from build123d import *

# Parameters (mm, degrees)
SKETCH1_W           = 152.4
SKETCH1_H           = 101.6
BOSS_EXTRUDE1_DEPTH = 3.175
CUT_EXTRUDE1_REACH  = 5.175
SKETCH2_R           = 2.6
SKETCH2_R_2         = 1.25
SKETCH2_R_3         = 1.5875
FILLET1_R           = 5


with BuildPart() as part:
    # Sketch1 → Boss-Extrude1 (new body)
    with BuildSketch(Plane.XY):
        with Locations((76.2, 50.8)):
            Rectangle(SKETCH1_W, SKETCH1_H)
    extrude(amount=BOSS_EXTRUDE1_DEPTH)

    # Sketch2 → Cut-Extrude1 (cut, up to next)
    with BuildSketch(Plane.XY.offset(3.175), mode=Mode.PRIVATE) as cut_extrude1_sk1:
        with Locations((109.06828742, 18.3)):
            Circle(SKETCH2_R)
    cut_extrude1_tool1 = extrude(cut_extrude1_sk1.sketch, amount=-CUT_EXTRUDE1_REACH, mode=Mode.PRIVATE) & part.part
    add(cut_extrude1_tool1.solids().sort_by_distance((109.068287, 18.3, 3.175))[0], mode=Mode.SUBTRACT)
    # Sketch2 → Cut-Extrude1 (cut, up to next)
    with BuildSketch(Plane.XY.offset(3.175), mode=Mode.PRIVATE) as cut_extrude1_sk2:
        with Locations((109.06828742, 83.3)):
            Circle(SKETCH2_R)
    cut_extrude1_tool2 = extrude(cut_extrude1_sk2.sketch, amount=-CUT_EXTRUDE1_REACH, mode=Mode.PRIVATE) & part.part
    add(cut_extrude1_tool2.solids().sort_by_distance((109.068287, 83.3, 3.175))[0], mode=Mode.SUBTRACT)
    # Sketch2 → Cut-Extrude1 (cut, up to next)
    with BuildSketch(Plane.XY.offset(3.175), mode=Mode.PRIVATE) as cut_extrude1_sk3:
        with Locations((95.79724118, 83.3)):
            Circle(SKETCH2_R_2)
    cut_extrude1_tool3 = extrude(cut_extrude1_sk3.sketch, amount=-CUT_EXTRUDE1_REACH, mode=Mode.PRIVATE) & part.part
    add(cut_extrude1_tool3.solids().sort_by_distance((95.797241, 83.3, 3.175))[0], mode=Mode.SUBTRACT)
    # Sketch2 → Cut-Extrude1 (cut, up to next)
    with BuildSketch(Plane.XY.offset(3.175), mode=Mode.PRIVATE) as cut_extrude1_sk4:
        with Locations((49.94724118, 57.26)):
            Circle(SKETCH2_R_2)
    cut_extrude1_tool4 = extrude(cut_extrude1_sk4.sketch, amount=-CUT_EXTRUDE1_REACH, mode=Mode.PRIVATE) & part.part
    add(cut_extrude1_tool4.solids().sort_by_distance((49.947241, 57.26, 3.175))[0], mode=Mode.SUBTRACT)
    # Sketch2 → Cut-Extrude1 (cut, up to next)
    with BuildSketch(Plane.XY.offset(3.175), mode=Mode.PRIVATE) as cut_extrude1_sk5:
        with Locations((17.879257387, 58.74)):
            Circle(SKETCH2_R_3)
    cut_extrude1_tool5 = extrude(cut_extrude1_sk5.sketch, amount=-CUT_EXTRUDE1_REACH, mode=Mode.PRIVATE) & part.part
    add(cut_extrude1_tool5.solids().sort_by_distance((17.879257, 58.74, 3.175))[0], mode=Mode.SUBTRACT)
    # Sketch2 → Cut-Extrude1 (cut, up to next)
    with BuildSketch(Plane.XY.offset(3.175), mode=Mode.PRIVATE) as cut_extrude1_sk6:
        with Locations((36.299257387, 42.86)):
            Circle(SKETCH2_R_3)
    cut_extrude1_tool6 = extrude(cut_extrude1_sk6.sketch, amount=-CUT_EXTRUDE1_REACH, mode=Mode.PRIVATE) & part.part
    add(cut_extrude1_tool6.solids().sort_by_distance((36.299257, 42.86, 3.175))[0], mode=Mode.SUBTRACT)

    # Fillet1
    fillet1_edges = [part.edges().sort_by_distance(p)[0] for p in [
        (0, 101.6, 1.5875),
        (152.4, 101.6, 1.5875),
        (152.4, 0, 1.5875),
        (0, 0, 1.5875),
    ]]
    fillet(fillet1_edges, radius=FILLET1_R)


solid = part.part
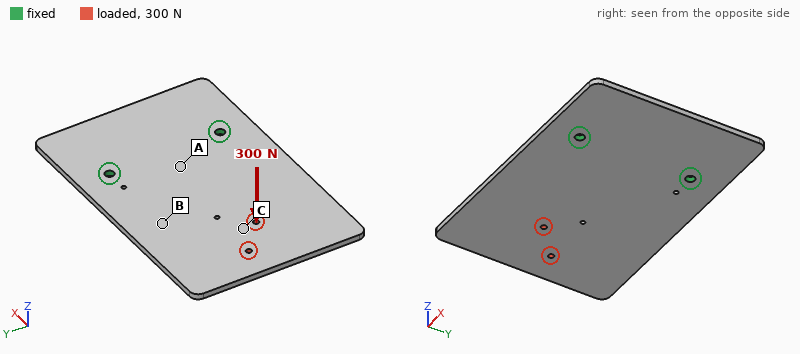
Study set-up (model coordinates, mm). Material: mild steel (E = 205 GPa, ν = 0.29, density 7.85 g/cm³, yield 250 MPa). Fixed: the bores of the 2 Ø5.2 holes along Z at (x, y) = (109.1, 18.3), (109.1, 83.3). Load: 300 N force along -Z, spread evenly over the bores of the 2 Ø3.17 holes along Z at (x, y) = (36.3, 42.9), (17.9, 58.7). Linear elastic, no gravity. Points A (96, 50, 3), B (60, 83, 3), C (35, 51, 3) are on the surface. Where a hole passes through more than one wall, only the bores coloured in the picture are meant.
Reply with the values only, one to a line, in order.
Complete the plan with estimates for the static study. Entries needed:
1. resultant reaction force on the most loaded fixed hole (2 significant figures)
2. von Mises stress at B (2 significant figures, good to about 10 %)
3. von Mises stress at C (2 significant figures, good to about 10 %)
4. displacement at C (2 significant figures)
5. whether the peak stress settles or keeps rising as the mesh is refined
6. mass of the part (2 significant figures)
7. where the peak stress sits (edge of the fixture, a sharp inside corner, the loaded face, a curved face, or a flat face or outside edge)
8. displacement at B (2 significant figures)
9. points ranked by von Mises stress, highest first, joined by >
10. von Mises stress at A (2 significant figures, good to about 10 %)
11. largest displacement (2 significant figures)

150 N
57 MPa
29 MPa
0.97 mm
keeps rising
380 g
edge of the fixture
0.48 mm
A > B > C
95 MPa
1.7 mm
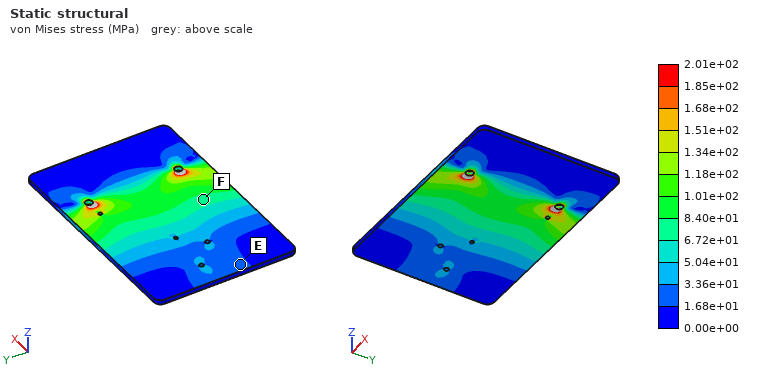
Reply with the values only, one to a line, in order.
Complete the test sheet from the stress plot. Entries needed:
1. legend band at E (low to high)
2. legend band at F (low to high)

1.68e+01 to 3.36e+01 MPa
6.72e+01 to 8.40e+01 MPa
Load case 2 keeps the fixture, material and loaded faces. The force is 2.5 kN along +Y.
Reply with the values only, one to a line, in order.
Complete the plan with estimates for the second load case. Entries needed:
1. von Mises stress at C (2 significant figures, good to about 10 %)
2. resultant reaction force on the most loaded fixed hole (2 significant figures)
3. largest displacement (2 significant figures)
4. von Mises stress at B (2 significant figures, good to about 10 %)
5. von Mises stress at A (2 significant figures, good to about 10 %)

19 MPa
3.3 kN
30 µm
15 MPa
16 MPa
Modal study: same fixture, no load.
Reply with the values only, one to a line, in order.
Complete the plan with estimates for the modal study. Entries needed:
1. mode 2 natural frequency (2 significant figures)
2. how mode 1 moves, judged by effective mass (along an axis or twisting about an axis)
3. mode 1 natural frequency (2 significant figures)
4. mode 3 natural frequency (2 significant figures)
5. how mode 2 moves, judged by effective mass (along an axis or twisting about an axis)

570 Hz
along Z
210 Hz
1200 Hz
twisting about X
